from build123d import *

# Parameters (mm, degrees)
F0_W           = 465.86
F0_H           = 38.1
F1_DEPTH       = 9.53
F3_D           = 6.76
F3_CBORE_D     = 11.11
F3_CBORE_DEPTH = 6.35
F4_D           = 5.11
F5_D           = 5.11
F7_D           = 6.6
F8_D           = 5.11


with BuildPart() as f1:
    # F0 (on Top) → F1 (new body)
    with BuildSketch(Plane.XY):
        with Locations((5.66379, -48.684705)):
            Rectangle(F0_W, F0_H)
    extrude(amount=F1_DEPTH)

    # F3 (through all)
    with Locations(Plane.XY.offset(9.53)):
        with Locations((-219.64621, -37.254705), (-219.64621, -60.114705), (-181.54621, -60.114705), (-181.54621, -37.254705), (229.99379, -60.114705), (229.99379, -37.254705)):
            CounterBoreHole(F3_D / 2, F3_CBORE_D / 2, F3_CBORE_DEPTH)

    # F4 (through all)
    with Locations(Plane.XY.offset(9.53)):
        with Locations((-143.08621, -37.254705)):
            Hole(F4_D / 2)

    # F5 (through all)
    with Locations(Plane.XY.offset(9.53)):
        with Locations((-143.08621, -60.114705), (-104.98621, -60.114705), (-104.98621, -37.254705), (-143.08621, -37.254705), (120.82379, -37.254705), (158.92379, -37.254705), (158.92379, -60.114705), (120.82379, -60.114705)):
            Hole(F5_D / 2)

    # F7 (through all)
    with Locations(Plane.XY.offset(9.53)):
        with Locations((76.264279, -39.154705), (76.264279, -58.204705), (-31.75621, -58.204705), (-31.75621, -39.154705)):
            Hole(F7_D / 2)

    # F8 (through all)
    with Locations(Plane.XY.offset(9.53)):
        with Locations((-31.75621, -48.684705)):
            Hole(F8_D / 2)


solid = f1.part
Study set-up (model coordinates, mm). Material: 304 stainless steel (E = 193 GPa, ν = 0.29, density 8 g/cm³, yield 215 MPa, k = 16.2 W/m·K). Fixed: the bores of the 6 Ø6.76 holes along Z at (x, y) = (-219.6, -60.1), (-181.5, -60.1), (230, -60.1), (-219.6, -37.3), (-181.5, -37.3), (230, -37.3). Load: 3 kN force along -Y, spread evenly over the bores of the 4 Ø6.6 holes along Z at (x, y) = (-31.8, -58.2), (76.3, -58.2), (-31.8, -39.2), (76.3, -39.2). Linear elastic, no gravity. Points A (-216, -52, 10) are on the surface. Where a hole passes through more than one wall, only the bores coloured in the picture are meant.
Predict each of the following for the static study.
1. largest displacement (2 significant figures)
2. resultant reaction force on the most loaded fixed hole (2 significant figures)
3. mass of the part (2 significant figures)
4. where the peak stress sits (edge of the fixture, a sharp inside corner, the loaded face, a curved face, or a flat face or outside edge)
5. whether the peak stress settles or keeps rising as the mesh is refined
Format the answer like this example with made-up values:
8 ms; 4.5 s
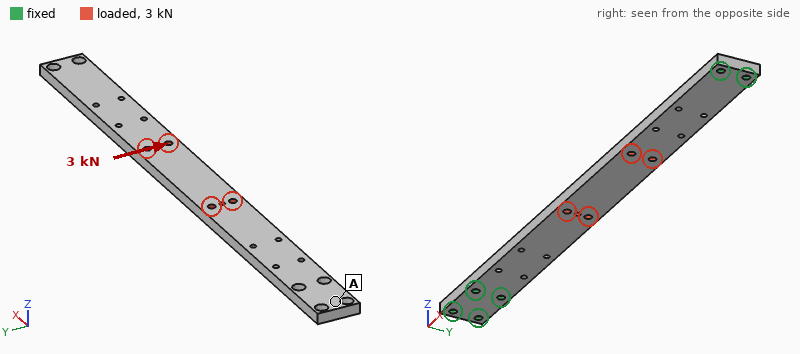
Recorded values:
0.14 mm; 5.0 kN; 1.3 kg; edge of the fixture; keeps rising
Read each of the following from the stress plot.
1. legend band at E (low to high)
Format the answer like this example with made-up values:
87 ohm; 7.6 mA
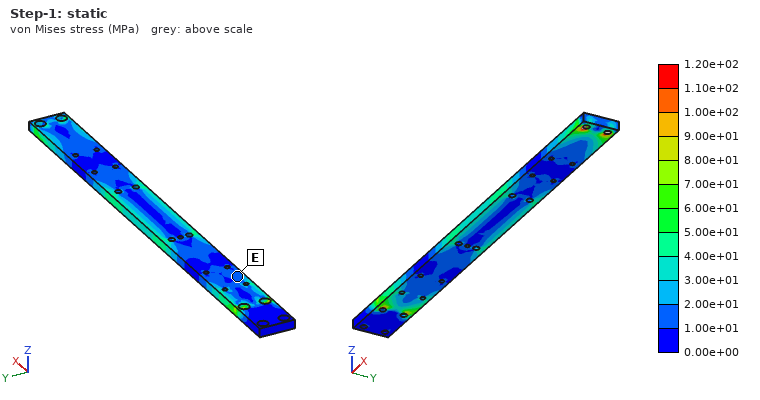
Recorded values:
1.00e+01 to 2.00e+01 MPa
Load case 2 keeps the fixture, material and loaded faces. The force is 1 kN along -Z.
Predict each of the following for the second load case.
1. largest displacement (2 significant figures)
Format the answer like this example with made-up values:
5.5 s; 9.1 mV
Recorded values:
0.70 mm
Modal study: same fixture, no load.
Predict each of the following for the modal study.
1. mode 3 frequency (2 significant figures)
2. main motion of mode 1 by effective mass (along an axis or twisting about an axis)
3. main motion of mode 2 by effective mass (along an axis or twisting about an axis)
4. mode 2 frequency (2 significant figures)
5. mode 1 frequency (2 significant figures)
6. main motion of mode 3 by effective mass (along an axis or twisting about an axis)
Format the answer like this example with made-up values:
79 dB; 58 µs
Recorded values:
980 Hz; along Z; twisting about Y; 700 Hz; 260 Hz; along Y
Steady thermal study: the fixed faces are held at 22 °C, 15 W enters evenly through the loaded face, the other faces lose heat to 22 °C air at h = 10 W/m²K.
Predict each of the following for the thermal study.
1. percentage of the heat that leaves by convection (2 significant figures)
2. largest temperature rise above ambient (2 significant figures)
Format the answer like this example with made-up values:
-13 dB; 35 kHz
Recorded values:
84 %; 63 K
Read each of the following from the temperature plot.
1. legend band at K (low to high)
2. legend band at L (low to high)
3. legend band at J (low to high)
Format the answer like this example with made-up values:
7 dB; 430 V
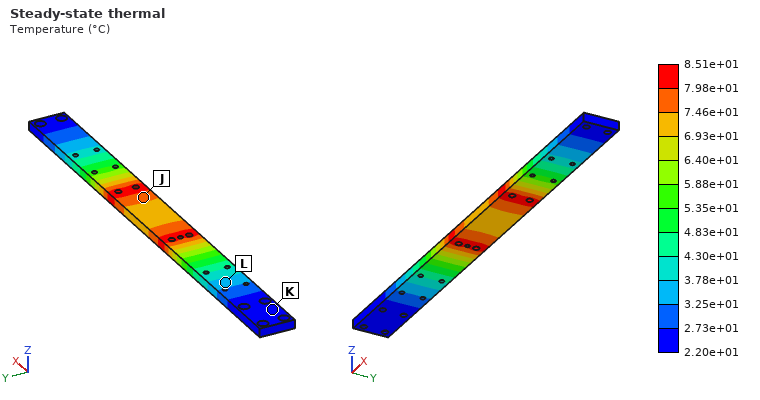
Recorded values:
2.20e+01 to 2.73e+01 °C; 3.25e+01 to 3.78e+01 °C; 7.46e+01 to 7.98e+01 °C
